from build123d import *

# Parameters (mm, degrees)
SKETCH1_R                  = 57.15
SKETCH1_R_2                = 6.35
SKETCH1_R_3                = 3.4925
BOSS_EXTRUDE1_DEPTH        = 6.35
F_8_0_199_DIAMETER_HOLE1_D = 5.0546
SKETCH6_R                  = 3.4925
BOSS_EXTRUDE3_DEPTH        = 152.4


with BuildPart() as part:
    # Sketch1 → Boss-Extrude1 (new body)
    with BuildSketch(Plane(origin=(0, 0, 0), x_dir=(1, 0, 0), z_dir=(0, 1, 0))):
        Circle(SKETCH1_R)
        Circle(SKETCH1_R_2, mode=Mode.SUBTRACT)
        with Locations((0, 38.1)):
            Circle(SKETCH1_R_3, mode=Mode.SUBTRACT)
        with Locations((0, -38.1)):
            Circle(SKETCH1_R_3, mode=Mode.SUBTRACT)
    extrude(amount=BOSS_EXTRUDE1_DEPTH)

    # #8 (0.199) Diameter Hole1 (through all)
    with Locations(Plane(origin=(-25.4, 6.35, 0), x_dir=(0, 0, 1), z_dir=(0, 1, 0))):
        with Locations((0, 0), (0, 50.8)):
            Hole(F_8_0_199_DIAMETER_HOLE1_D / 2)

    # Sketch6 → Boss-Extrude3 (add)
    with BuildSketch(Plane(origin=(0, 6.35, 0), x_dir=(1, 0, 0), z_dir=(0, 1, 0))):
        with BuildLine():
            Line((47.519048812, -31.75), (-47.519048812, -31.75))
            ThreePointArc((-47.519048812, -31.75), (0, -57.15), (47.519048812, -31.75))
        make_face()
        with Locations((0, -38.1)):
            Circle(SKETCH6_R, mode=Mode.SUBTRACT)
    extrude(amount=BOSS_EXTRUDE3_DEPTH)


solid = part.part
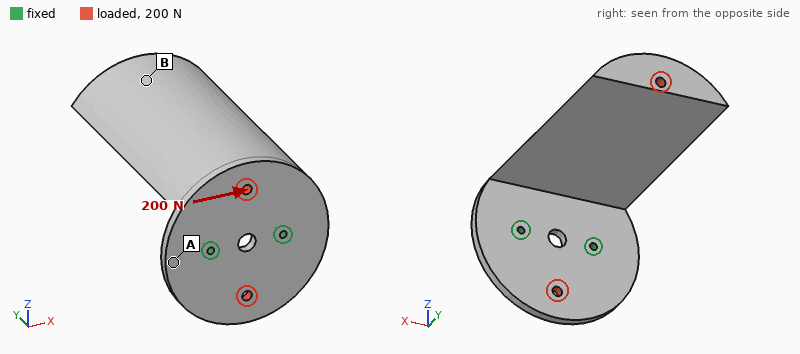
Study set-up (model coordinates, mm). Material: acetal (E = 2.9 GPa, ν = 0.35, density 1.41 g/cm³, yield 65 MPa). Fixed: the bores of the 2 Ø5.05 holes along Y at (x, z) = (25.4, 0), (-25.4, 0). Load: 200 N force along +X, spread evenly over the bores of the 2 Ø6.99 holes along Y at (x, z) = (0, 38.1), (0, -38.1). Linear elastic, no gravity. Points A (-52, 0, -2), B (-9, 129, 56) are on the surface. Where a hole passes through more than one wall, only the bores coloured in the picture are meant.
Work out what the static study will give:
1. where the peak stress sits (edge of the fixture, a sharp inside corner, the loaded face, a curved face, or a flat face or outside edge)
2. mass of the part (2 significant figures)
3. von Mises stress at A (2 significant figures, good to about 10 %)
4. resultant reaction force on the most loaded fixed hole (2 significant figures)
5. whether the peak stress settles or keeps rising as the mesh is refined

edge of the fixture
450 g
4.6 MPa
290 N
keeps rising
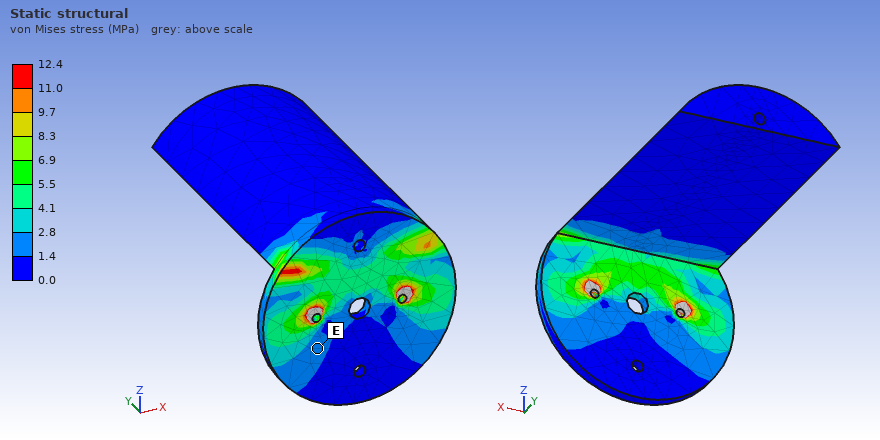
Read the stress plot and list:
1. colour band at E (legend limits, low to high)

1.4 to 2.8 MPa
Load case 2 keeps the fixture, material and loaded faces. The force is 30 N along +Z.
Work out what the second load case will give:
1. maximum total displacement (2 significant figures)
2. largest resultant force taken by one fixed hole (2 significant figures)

2.2 mm
15 N
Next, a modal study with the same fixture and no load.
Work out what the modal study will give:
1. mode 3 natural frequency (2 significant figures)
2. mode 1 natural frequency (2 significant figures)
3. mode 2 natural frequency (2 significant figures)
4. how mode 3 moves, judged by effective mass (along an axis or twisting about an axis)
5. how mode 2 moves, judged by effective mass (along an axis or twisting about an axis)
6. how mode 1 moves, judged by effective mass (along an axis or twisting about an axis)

270 Hz
36 Hz
91 Hz
along Y
along X
along Z
